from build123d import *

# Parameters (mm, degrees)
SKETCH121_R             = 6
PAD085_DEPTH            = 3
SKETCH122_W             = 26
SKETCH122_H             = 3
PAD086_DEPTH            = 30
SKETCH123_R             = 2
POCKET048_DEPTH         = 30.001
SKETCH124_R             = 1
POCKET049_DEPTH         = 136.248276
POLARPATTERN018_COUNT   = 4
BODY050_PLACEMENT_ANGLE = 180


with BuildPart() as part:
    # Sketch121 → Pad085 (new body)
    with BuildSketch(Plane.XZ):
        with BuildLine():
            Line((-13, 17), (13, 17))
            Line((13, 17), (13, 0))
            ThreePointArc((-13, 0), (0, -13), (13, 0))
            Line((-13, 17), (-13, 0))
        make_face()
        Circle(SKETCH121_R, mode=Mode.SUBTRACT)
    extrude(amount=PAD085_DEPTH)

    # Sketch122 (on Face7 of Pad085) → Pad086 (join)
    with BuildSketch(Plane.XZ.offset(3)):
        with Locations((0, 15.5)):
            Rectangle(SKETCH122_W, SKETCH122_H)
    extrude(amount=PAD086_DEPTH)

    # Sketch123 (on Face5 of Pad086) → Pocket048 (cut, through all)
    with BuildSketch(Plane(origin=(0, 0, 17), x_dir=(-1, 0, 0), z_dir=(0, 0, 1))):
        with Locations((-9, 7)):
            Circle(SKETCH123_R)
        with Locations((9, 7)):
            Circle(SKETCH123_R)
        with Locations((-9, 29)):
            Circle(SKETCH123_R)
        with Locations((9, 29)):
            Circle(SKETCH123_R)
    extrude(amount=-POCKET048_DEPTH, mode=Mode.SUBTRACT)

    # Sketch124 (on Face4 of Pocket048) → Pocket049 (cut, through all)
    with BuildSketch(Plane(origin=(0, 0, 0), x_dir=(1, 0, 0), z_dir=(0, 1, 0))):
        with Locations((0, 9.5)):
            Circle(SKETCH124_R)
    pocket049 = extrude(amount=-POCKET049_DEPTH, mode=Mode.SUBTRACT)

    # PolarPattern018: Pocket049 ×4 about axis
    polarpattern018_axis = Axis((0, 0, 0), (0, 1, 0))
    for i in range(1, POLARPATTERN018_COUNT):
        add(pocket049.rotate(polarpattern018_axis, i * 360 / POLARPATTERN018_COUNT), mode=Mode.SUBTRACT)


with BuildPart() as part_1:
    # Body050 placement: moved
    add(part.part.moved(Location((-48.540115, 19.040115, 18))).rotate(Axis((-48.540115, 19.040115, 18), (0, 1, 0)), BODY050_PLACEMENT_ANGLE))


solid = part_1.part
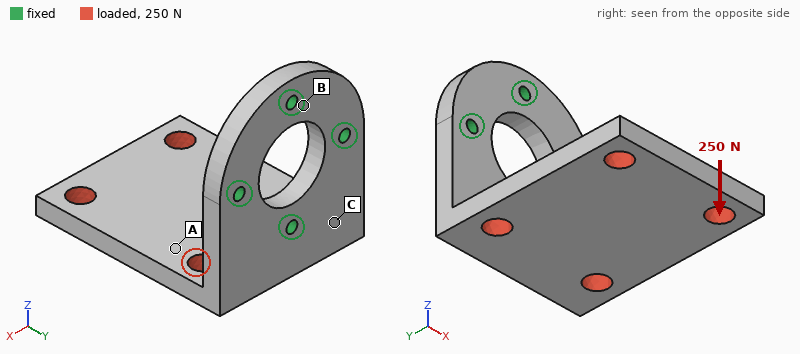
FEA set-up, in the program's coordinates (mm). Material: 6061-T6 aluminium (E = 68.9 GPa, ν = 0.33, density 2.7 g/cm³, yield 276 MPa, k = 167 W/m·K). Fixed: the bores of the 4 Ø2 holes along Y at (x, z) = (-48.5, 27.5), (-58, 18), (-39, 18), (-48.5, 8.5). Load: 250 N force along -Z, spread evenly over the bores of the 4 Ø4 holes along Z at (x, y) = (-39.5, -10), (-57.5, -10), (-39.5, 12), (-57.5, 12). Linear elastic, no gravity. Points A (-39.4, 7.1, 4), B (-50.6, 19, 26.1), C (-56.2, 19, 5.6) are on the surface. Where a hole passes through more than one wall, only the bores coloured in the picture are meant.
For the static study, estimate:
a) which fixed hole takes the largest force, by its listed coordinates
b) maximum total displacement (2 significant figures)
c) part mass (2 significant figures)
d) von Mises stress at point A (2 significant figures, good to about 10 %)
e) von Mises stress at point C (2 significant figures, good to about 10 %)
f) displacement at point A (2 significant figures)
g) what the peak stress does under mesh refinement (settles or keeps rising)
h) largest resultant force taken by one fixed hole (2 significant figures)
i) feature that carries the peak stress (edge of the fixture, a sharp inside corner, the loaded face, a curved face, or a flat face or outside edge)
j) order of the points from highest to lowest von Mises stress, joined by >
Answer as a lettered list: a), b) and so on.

a) (-48.5, 8.5)
b) 0.51 mm
c) 11 g
d) 45 MPa
e) 79 MPa
f) 0.12 mm
g) keeps rising
h) 280 N
i) edge of the fixture
j) C > A > B
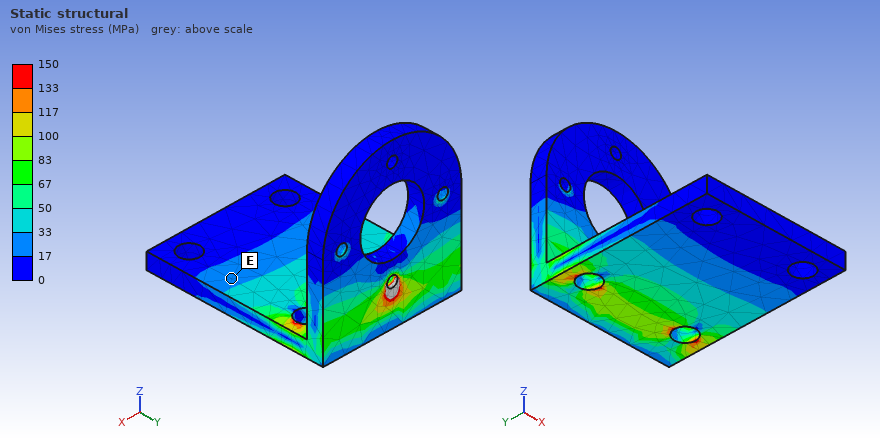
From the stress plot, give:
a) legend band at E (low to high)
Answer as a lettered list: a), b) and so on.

a) 17 to 33 MPa
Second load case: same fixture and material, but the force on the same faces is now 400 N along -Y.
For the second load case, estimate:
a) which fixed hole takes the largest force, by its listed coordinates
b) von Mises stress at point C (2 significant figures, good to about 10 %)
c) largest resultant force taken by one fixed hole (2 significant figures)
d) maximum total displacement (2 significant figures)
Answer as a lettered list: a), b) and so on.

a) (-48.5, 8.5)
b) 20 MPa
c) 470 N
d) 93 µm
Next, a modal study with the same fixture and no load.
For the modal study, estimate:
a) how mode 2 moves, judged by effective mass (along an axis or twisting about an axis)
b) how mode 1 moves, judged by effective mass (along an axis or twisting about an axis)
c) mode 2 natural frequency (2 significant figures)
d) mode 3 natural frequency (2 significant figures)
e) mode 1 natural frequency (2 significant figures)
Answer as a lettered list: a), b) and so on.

a) along X
b) along Z
c) 3100 Hz
d) 6400 Hz
e) 1800 Hz
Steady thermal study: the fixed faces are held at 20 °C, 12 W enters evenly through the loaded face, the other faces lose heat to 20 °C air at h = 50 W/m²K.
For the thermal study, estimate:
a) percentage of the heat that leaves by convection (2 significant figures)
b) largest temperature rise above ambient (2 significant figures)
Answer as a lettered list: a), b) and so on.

a) 13 %
b) 23 K
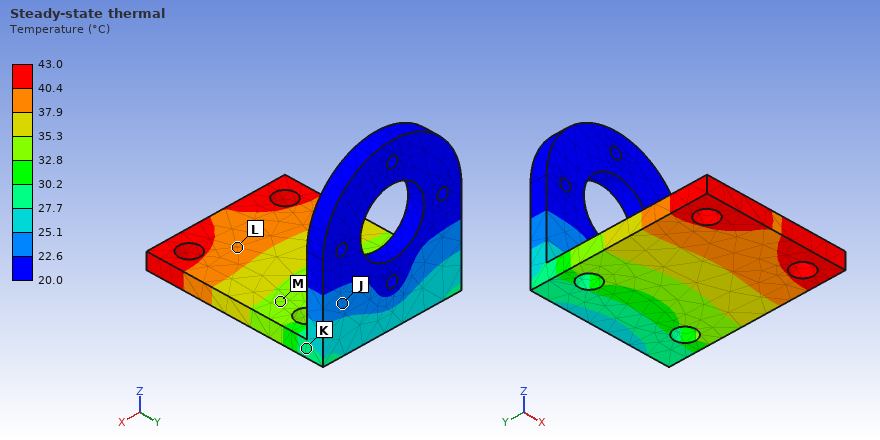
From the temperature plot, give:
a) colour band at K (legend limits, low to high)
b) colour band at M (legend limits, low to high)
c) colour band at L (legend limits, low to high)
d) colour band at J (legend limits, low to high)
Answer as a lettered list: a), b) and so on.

a) 27.7 to 30.2 °C
b) 32.8 to 35.3 °C
c) 37.9 to 40.4 °C
d) 22.6 to 25.1 °C
